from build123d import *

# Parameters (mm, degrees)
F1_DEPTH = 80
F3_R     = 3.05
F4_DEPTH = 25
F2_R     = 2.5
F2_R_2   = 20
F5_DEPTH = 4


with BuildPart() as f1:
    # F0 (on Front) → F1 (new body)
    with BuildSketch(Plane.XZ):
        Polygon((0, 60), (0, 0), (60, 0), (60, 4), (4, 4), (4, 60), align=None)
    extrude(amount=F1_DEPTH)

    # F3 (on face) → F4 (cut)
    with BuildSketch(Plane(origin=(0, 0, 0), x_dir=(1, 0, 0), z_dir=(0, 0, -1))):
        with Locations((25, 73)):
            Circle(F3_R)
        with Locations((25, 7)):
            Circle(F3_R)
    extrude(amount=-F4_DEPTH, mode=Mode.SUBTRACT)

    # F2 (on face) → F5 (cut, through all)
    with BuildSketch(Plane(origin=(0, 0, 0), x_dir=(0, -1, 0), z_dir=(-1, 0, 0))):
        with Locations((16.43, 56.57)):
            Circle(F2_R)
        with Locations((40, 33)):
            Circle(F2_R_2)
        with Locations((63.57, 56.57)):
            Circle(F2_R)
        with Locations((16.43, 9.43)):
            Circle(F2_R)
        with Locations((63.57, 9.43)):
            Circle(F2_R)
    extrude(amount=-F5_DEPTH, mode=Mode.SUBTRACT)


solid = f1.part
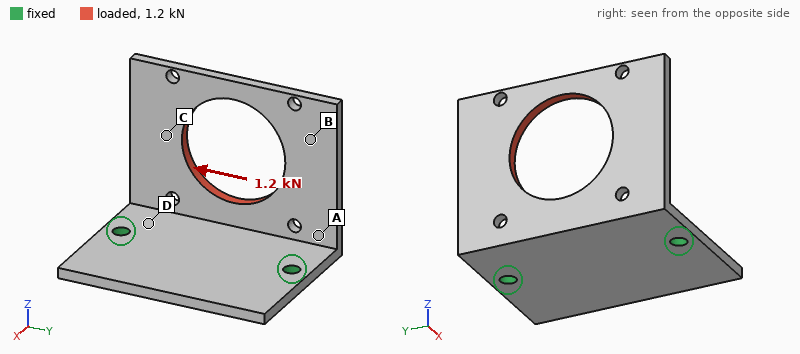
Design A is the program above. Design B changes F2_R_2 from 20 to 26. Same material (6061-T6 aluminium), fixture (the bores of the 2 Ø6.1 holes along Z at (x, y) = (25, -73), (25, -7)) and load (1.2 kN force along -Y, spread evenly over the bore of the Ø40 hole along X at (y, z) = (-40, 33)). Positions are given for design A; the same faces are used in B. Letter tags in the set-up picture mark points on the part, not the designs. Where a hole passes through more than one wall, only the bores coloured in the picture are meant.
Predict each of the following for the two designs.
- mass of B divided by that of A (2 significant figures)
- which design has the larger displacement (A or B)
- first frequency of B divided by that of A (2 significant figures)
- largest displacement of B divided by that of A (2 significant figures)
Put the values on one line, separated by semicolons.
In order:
0.89; B; 1.1; 1.4
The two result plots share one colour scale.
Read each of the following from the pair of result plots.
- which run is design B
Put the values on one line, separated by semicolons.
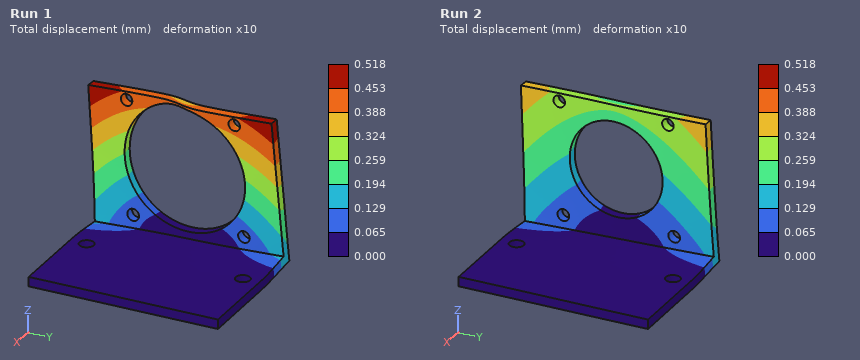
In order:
Run 1
